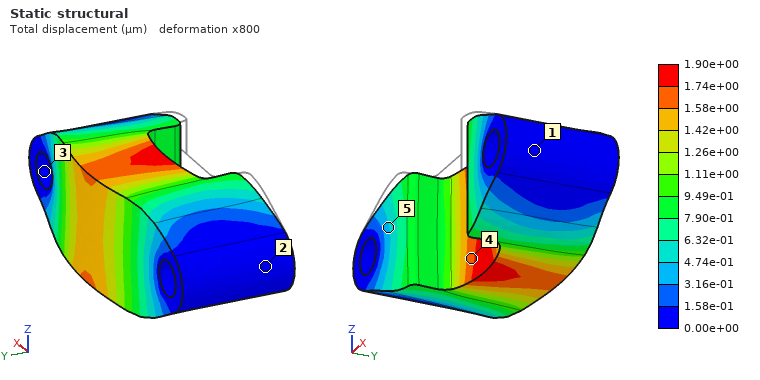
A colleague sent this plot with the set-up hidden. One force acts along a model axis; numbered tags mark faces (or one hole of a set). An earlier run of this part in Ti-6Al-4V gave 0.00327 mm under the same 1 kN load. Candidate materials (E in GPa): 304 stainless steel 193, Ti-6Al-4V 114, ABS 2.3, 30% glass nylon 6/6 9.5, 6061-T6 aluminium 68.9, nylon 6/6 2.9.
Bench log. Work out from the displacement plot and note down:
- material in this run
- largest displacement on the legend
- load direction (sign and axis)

304 stainless steel
1.90e+00 µm
+Y
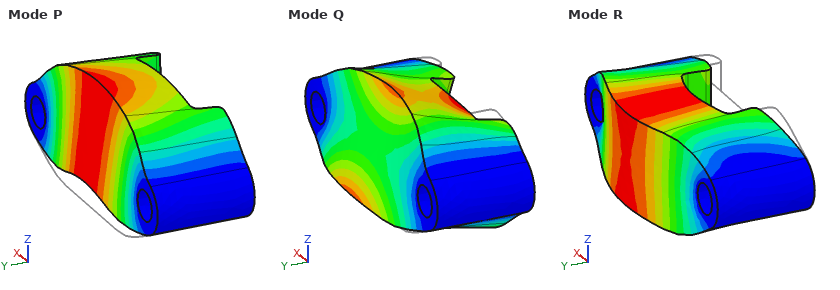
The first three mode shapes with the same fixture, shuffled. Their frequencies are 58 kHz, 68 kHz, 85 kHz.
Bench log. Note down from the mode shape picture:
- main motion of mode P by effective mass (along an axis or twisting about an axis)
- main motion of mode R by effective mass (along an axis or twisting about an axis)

along Z
along Y
